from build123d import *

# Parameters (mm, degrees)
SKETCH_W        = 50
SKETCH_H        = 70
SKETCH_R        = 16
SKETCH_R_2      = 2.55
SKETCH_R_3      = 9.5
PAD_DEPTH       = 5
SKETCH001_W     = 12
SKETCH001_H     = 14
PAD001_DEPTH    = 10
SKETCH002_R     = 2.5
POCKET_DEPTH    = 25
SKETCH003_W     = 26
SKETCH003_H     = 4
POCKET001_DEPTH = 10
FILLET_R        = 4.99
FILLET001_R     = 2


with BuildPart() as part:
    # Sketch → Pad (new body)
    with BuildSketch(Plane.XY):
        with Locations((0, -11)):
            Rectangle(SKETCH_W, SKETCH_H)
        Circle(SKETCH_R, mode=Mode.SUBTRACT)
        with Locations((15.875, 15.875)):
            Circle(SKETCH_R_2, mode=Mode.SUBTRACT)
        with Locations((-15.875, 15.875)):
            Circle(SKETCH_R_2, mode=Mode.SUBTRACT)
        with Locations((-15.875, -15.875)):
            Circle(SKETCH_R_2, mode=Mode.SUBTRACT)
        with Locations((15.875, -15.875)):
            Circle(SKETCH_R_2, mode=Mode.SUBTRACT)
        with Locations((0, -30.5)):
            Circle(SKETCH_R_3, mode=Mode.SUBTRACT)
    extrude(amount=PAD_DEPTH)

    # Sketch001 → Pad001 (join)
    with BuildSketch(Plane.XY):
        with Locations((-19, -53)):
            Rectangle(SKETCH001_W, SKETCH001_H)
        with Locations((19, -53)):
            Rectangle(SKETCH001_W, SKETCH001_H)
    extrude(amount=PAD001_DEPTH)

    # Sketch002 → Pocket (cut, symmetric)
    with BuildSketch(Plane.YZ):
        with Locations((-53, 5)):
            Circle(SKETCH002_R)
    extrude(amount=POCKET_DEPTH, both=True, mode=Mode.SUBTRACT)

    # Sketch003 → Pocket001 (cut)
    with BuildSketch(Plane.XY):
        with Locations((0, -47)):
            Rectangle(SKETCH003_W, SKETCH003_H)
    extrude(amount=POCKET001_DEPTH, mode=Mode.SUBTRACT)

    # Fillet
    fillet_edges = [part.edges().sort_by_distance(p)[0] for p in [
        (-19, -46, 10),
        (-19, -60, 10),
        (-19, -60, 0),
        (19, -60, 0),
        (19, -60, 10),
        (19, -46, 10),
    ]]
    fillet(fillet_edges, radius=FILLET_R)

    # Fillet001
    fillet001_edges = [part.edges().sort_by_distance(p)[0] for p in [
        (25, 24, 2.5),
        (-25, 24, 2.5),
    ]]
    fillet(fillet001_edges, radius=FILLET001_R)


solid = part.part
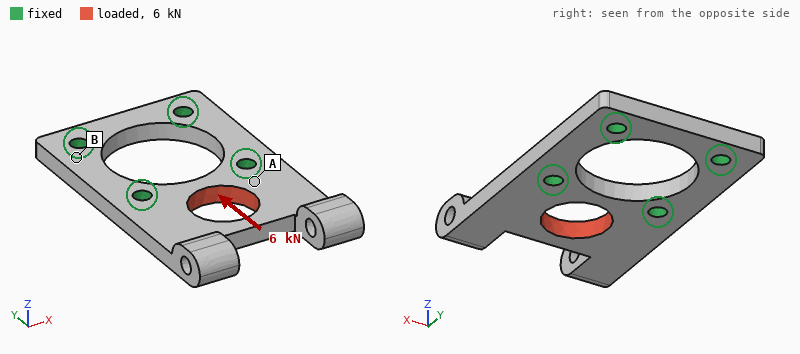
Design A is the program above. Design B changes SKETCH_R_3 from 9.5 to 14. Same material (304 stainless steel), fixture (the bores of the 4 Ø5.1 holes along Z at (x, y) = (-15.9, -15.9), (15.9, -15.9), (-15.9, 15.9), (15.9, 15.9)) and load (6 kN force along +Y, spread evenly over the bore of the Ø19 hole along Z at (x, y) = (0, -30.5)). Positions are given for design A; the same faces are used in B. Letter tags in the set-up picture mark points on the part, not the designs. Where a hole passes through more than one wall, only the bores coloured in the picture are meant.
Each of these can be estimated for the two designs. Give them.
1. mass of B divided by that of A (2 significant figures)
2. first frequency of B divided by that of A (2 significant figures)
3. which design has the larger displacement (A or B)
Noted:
0.88
0.89
B
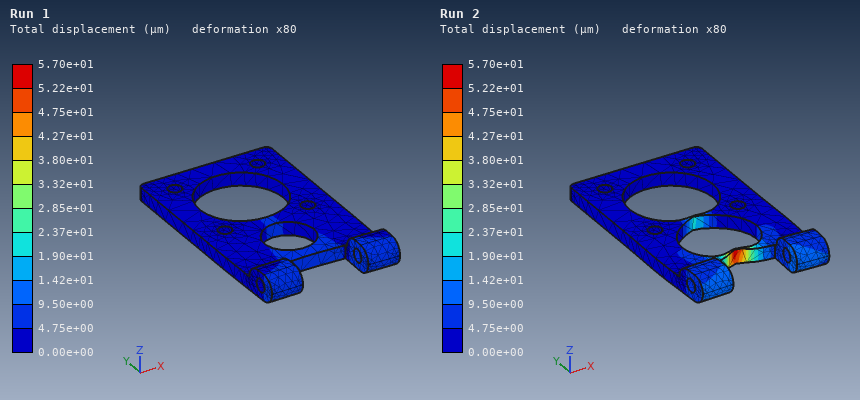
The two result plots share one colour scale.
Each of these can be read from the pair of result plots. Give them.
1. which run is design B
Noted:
Run 2
